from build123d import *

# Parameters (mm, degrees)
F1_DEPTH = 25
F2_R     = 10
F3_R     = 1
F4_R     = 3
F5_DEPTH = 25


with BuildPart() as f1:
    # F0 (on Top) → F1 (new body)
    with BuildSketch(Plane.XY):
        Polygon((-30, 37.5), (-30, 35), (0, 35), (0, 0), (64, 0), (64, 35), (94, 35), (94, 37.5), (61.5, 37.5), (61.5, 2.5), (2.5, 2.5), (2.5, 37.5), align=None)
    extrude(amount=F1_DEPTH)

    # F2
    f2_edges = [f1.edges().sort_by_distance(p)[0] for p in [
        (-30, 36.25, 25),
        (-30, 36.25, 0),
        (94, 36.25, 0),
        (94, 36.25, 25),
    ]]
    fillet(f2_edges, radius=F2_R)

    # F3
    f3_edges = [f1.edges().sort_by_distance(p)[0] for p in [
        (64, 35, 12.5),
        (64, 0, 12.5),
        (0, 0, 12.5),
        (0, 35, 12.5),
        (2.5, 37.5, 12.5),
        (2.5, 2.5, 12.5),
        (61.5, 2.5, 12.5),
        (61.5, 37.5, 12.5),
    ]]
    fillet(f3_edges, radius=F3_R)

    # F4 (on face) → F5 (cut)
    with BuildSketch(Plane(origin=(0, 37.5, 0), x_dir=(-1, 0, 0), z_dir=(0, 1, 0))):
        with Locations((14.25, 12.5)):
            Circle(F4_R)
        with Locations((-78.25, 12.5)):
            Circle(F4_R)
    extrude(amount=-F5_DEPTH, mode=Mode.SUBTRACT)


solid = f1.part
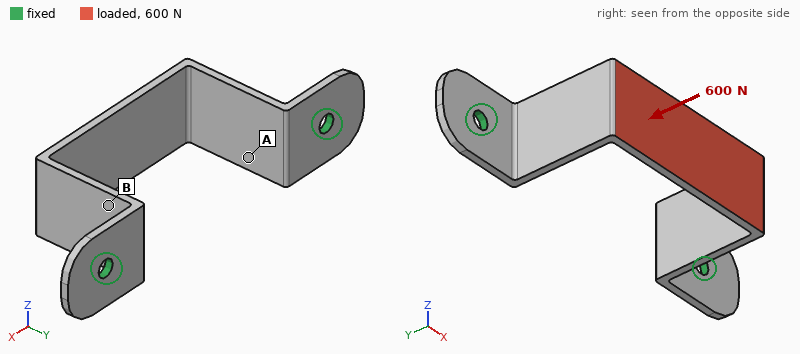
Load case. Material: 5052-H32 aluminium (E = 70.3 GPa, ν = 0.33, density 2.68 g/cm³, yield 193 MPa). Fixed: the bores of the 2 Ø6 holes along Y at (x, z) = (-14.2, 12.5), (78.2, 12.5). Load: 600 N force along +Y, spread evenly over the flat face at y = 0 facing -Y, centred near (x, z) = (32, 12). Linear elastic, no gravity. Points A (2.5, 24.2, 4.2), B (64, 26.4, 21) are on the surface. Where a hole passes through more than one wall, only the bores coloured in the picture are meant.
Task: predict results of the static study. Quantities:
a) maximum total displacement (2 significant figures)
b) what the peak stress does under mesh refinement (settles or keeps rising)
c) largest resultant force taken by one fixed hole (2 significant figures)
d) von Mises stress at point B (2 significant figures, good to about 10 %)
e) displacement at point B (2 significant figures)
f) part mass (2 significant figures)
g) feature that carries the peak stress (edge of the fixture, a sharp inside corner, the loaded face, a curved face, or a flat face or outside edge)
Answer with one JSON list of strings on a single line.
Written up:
["0.31 mm", "keeps rising", "330 N", "27 MPa", "0.050 mm", "32 g", "edge of the fixture"]
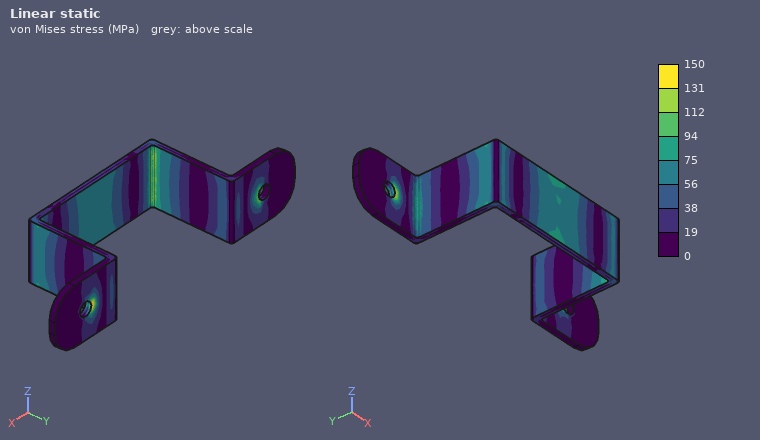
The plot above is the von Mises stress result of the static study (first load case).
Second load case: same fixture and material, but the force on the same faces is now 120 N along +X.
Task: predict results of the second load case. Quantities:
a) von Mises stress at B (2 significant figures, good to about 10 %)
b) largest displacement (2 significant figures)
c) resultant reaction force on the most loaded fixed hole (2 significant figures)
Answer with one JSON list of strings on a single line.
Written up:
["16 MPa", "0.21 mm", "71 N"]
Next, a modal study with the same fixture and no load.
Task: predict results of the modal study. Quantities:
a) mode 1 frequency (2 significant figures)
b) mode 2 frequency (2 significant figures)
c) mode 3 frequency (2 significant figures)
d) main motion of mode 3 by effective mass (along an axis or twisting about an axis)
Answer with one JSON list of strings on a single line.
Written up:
["950 Hz", "980 Hz", "1600 Hz", "twisting about Y"]
